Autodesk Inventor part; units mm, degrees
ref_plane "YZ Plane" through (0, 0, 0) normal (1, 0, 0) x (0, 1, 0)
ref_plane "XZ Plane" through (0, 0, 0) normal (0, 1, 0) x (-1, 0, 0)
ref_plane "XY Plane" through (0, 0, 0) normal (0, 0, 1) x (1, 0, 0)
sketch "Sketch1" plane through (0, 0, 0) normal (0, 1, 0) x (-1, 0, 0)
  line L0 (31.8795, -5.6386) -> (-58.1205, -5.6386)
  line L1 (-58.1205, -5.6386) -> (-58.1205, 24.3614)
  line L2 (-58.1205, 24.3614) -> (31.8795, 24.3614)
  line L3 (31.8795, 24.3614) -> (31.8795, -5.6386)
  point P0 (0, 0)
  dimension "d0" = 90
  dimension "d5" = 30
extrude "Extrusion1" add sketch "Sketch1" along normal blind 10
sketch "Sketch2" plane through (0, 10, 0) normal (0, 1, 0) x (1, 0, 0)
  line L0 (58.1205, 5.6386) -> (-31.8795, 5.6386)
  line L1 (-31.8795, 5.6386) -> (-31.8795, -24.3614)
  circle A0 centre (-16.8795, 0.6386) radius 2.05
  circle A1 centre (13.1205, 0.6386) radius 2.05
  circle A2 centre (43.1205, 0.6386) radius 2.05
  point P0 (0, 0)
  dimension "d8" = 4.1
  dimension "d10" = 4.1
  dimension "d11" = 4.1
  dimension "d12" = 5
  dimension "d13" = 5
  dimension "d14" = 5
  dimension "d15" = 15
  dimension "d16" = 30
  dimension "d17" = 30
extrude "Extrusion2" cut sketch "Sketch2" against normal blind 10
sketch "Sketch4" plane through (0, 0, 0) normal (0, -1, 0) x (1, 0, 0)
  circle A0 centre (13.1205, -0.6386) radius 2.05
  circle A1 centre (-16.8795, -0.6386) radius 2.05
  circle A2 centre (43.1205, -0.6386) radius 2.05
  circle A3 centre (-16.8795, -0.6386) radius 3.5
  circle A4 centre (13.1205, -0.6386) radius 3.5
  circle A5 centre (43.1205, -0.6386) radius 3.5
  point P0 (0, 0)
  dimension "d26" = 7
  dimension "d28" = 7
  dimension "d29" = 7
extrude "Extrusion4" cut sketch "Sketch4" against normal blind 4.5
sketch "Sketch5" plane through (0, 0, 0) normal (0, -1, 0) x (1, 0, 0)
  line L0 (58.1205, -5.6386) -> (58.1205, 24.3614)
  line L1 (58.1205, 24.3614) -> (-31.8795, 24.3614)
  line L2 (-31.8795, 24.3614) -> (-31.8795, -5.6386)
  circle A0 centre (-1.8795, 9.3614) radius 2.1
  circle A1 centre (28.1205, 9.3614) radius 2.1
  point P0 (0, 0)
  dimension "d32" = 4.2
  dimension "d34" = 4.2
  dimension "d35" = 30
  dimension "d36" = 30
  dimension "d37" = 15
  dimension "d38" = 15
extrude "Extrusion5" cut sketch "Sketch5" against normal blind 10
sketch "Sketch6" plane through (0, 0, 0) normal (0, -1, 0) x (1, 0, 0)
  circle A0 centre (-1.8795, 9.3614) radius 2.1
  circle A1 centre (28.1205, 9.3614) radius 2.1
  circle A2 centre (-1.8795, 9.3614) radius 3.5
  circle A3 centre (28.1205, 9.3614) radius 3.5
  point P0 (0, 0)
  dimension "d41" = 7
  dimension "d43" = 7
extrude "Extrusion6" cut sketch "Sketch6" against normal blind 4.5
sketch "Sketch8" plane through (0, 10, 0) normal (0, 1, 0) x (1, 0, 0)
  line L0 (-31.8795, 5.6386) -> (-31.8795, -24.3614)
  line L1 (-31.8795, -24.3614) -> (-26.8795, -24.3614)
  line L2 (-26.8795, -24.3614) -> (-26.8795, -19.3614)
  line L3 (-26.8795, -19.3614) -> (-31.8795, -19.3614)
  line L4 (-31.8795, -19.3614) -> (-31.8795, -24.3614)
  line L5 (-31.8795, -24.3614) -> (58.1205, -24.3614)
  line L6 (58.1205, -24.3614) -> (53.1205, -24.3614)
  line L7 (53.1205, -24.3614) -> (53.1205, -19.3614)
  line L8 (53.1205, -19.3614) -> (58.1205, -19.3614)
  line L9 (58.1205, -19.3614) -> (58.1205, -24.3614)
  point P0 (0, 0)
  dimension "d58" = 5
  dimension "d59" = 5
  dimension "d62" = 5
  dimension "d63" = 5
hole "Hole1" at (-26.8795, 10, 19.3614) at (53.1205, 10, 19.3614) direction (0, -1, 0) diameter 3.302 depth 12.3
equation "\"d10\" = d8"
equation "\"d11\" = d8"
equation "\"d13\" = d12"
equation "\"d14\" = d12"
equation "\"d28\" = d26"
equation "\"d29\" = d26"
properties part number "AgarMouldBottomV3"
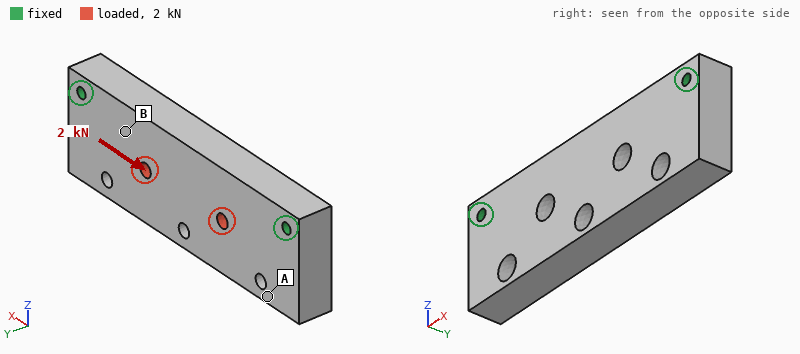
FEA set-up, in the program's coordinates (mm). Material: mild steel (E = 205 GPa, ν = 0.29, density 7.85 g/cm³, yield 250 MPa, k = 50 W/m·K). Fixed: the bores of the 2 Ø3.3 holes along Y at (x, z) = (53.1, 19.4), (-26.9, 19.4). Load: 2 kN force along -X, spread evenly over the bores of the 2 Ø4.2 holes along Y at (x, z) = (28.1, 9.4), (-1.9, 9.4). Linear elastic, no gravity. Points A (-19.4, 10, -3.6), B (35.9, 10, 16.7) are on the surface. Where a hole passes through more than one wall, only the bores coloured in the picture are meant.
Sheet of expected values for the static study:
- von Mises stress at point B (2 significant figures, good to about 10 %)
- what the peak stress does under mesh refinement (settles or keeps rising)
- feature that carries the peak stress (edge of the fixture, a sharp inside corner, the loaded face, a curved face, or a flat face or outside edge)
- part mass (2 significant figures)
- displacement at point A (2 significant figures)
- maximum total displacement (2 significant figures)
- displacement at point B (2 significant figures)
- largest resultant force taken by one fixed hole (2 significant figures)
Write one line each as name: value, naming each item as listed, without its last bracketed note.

von Mises stress at point B: 7.2 MPa
what the peak stress does under mesh refinement: keeps rising
feature that carries the peak stress: edge of the fixture
part mass: 200 g
displacement at point A: 1.0 µm
maximum total displacement: 1.4 µm
displacement at point B: 0.71 µm
largest resultant force taken by one fixed hole: 1.0 kN
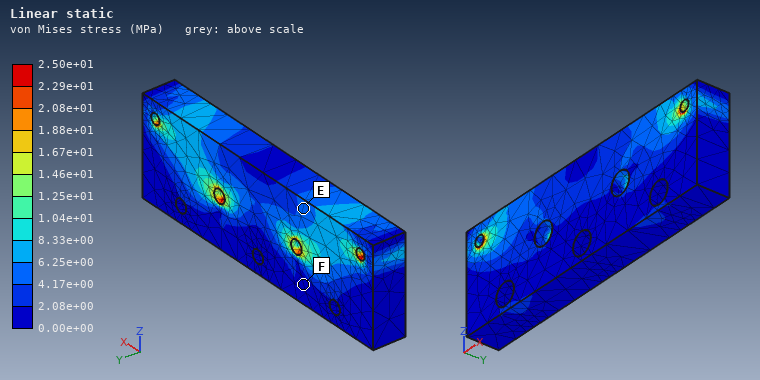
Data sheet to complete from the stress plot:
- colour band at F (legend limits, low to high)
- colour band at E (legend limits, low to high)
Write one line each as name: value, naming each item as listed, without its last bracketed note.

colour band at F: 0.00e+00 to 2.08e+00 MPa
colour band at E: 4.17e+00 to 6.25e+00 MPa
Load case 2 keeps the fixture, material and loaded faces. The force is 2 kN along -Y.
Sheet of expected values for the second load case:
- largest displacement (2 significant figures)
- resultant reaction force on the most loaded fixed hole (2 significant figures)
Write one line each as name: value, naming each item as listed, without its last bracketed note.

largest displacement: 24 µm
resultant reaction force on the most loaded fixed hole: 1.0 kN
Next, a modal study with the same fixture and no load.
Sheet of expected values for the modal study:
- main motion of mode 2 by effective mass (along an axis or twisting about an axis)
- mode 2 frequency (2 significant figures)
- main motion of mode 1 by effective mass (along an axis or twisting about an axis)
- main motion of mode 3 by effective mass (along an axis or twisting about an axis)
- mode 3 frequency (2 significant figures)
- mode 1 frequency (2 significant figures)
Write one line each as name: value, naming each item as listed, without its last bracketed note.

main motion of mode 2 by effective mass: twisting about X
mode 2 frequency: 8900 Hz
main motion of mode 1 by effective mass: along Y
main motion of mode 3 by effective mass: along Z
mode 3 frequency: 11 kHz
mode 1 frequency: 4800 Hz
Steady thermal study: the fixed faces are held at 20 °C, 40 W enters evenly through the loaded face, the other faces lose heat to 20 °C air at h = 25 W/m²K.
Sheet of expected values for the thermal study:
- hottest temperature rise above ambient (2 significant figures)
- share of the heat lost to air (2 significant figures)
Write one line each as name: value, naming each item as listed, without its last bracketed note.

hottest temperature rise above ambient: 57 K
share of the heat lost to air: 15 %
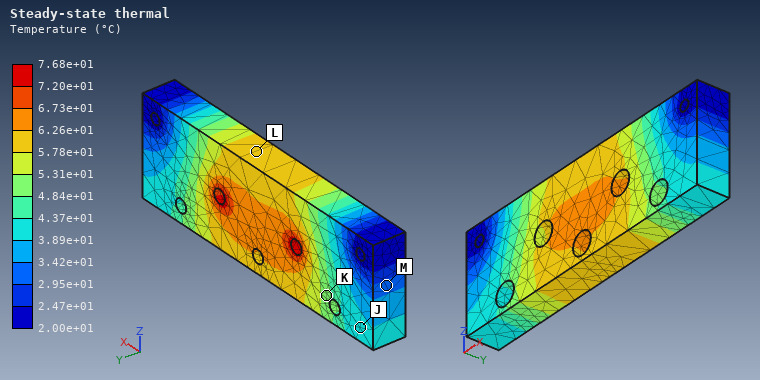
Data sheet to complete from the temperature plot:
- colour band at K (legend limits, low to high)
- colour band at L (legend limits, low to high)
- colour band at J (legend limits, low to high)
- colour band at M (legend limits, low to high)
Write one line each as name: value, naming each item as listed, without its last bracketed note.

colour band at K: 4.84e+01 to 5.31e+01 °C
colour band at L: 5.78e+01 to 6.26e+01 °C
colour band at J: 3.89e+01 to 4.37e+01 °C
colour band at M: 2.95e+01 to 3.42e+01 °C
